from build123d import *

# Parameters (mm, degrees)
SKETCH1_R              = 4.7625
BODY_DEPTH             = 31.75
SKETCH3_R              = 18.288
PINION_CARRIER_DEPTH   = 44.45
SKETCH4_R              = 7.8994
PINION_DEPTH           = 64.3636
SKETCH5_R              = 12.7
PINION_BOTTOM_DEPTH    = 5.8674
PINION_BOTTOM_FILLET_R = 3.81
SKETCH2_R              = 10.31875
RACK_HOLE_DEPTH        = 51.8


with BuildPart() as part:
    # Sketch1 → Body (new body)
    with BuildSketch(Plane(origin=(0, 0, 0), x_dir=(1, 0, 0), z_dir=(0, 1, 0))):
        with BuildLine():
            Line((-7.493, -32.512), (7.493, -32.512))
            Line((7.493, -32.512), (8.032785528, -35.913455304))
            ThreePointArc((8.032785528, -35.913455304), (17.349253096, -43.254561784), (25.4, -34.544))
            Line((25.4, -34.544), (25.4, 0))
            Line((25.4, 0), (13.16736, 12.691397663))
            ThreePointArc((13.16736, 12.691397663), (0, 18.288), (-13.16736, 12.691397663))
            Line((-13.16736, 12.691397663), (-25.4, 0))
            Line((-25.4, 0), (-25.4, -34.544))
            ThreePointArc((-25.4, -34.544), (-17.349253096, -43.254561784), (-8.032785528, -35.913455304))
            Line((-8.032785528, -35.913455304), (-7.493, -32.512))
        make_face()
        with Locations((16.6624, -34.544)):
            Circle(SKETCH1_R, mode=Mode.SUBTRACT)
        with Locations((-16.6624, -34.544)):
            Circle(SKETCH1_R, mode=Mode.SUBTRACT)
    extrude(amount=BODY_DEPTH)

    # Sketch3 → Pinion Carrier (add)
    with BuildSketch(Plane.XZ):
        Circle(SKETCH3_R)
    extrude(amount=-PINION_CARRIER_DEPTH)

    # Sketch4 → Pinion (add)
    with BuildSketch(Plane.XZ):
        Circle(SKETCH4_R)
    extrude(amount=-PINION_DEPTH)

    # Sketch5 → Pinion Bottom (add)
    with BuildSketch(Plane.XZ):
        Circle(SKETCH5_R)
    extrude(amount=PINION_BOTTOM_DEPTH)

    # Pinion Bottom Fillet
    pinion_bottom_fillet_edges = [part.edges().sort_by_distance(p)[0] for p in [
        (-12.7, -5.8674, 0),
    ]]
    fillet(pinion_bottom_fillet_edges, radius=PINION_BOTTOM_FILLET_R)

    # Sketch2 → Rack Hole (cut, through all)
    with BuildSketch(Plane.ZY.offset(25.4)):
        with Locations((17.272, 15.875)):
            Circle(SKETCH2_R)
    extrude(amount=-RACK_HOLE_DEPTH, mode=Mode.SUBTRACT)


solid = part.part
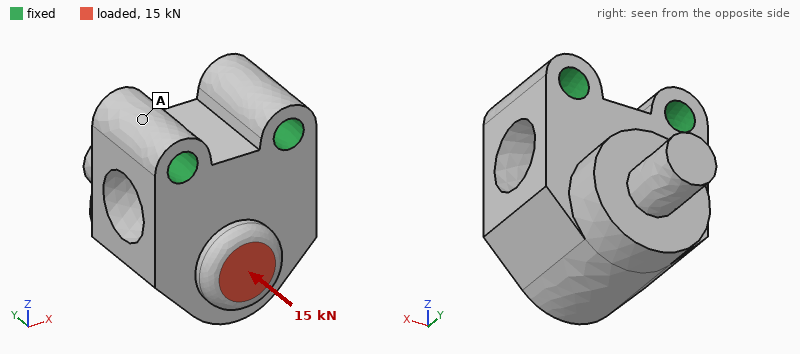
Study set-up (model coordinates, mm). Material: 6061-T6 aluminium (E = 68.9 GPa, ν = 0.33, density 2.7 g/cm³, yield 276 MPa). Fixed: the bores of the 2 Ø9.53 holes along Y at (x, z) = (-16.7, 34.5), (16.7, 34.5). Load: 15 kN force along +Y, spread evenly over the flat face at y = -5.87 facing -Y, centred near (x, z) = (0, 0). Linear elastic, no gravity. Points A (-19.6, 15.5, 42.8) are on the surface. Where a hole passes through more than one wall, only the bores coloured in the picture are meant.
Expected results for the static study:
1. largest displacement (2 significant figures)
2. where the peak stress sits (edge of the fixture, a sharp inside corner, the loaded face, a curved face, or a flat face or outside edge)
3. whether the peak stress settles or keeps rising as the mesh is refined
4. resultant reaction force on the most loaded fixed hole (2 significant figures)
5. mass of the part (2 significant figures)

0.15 mm
edge of the fixture
keeps rising
7.5 kN
210 g
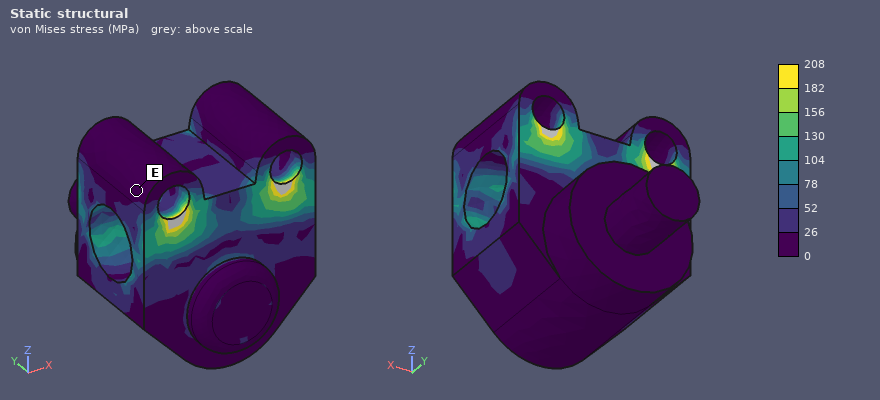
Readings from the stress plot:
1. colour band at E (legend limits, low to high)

0 to 26 MPa
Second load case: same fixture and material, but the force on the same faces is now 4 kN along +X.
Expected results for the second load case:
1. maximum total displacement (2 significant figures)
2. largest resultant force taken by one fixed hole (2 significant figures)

29 µm
4.1 kN
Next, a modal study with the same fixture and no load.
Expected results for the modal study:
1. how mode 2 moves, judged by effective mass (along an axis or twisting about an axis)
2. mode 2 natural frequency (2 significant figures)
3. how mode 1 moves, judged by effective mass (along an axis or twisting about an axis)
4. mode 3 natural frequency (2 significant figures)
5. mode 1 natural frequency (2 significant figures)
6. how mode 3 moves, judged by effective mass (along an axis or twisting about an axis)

along X
6800 Hz
along Y
8900 Hz
4700 Hz
along X
